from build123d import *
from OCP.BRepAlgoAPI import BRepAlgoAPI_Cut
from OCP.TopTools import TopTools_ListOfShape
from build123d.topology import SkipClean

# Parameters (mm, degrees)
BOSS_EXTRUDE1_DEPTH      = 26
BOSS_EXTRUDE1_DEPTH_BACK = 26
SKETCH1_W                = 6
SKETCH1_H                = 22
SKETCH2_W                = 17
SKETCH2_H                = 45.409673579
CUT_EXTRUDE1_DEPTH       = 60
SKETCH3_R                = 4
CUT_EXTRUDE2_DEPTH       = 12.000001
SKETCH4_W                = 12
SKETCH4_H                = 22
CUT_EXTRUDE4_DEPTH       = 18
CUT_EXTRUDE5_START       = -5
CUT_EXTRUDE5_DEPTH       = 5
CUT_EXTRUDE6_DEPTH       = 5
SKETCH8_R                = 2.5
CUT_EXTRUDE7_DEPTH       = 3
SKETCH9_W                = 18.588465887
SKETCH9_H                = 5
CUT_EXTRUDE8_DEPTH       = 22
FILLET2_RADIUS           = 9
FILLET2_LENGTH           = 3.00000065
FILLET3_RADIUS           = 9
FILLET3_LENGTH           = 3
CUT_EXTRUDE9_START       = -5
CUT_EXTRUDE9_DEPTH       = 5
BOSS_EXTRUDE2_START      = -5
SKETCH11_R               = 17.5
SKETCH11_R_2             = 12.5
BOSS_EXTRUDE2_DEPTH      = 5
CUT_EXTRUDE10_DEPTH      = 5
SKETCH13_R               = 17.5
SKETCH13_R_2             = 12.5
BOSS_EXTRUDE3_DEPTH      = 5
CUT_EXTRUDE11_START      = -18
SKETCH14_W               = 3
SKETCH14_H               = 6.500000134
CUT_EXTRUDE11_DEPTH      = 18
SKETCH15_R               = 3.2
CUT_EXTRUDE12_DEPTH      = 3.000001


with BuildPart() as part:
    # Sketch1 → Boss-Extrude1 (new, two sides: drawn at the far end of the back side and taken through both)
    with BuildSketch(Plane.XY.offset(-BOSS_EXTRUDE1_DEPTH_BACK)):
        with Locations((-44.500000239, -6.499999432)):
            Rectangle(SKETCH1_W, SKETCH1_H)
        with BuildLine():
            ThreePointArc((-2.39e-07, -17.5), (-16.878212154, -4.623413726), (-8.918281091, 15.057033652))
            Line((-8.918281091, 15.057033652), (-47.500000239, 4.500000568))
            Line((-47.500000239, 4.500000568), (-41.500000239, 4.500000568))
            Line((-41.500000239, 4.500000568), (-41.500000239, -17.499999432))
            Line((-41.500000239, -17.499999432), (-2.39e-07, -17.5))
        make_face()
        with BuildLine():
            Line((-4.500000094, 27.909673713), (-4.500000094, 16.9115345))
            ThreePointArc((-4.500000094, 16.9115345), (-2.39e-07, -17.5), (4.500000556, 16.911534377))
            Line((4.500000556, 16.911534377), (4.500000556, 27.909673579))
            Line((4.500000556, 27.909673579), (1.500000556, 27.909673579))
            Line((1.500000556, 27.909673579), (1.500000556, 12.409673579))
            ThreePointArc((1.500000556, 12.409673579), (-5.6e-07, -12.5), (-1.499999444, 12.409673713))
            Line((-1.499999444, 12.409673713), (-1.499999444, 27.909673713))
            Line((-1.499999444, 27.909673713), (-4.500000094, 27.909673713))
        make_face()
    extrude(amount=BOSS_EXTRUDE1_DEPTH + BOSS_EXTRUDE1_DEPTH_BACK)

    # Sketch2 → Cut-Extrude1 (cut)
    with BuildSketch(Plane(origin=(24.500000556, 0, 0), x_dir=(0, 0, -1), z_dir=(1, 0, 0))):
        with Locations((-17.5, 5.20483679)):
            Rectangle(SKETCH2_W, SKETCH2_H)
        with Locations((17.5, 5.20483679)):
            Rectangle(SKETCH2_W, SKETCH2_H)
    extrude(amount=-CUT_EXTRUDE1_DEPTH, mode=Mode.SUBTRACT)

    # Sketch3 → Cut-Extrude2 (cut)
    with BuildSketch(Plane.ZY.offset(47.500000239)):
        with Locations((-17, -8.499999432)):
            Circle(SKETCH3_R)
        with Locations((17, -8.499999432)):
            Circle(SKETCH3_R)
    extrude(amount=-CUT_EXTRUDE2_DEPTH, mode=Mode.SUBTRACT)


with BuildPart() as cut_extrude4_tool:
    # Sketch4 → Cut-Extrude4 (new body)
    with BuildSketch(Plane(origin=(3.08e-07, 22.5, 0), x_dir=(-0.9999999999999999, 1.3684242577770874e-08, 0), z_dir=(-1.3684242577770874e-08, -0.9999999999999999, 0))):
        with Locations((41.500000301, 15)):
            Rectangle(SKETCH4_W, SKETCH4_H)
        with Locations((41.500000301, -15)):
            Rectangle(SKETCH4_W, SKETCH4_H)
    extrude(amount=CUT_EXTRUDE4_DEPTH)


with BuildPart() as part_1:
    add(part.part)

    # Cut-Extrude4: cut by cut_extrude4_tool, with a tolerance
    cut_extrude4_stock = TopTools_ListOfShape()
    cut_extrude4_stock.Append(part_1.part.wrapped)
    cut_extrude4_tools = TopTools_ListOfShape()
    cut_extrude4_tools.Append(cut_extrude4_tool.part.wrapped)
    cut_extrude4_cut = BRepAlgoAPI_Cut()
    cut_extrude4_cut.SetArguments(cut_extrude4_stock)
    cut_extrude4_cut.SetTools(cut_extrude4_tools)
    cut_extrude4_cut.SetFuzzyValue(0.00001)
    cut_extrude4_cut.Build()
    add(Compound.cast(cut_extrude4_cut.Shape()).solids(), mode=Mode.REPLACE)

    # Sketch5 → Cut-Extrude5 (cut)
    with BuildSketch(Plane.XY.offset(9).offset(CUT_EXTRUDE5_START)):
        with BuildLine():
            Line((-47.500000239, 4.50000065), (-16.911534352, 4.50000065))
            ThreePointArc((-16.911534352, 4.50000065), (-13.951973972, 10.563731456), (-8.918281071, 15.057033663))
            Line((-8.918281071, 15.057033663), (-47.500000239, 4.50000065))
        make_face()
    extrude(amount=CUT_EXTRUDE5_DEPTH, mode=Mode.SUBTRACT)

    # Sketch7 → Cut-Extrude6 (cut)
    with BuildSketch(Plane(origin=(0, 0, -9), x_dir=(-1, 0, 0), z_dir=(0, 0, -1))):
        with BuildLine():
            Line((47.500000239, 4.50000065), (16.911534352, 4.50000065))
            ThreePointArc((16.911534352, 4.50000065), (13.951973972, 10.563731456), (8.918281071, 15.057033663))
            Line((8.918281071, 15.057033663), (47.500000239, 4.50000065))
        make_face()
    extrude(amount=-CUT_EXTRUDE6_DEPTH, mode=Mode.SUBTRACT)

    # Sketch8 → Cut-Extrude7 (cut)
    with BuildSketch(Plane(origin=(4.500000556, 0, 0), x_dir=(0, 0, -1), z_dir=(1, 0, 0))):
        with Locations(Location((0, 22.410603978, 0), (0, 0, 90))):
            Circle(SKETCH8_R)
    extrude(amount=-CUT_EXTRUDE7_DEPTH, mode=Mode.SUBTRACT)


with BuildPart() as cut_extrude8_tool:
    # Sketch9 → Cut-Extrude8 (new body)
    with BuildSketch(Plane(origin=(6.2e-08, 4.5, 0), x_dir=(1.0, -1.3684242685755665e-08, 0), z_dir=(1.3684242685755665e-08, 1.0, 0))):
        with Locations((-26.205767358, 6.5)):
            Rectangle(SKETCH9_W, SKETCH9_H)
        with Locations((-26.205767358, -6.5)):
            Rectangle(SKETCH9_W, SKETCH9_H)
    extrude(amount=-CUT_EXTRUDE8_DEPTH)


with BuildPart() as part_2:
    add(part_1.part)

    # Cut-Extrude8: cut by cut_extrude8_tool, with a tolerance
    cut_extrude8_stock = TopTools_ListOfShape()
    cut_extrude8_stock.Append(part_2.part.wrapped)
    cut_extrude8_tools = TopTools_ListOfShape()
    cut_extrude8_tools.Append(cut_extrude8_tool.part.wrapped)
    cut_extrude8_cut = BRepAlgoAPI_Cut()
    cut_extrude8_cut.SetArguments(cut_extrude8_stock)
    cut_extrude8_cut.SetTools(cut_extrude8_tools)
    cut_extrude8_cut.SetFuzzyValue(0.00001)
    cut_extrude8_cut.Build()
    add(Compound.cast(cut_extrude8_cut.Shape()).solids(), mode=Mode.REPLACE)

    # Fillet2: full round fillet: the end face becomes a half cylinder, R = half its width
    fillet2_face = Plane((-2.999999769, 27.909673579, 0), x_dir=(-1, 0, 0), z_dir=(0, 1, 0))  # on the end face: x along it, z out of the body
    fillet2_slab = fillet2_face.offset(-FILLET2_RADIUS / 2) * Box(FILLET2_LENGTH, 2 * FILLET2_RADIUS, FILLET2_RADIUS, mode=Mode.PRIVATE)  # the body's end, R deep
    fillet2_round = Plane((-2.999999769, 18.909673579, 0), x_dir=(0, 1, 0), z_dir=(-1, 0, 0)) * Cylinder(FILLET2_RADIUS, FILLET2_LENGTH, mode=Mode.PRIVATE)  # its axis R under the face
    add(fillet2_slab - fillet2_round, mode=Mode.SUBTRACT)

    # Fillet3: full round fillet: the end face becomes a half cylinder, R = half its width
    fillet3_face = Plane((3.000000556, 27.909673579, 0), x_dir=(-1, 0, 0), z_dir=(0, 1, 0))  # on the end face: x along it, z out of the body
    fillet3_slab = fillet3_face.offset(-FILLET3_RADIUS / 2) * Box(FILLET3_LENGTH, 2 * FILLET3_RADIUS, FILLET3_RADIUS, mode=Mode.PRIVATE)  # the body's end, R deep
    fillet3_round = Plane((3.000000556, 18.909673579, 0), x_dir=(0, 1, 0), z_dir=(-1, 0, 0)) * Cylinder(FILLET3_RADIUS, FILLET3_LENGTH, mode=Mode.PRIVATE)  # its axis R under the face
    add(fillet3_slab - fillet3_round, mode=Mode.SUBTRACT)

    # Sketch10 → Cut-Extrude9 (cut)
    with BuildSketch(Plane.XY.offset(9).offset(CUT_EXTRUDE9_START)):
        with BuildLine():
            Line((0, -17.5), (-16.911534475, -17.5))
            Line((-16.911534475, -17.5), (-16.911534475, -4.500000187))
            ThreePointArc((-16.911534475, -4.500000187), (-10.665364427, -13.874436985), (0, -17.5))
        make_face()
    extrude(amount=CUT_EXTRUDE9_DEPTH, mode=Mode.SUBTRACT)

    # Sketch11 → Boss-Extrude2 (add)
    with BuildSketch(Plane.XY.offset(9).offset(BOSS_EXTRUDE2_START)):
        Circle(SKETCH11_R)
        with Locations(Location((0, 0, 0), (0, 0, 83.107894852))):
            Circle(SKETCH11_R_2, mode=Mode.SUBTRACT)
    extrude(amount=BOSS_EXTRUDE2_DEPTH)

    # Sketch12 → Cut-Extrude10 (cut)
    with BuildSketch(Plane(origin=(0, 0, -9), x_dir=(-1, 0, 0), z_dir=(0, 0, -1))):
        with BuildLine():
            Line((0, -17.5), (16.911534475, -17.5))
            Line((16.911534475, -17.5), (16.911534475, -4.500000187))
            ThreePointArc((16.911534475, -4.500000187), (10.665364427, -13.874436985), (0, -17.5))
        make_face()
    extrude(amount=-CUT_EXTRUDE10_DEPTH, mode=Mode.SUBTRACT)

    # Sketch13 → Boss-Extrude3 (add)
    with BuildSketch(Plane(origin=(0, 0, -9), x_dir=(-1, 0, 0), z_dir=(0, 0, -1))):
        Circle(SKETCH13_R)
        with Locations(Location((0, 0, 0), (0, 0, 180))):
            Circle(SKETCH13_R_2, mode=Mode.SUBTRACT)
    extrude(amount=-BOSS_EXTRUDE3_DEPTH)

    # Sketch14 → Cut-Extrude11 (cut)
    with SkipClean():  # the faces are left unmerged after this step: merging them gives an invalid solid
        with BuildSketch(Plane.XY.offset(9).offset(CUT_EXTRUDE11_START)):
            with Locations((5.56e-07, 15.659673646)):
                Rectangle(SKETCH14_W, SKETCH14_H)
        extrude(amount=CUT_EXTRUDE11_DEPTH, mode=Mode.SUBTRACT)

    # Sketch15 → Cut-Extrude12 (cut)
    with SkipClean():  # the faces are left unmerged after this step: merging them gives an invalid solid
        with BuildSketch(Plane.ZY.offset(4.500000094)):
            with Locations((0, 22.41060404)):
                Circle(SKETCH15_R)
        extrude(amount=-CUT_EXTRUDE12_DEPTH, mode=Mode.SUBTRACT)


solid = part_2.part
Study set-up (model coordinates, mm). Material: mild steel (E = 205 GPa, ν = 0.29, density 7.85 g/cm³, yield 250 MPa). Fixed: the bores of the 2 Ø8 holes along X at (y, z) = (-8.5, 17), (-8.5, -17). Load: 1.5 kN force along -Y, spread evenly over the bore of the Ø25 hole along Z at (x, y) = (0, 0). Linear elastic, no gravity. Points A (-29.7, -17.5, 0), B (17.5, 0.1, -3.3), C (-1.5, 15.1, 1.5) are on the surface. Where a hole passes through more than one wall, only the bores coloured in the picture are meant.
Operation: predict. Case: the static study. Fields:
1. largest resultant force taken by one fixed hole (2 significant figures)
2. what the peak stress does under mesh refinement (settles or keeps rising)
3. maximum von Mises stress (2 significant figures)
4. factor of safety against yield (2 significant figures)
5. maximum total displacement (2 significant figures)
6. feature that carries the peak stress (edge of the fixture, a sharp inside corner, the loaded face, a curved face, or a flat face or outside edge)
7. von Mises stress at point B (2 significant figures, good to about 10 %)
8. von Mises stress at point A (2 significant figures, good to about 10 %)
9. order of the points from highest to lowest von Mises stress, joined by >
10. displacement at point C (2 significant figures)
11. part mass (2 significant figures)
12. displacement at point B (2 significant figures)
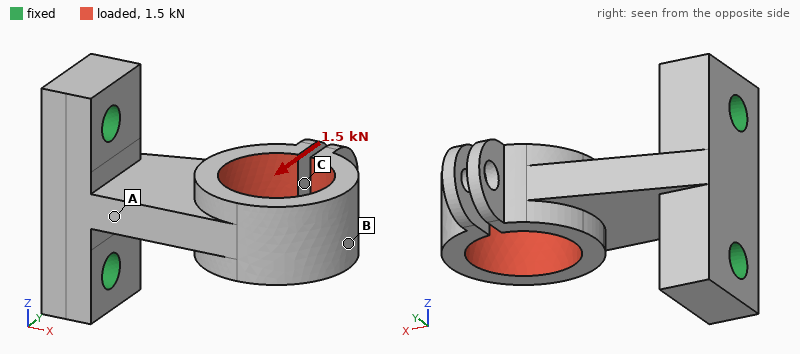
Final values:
780 N
settles
140 MPa
1.8
0.16 mm
a flat face or outside edge
22 MPa
55 MPa
A > B > C
0.042 mm
210 g
0.13 mm
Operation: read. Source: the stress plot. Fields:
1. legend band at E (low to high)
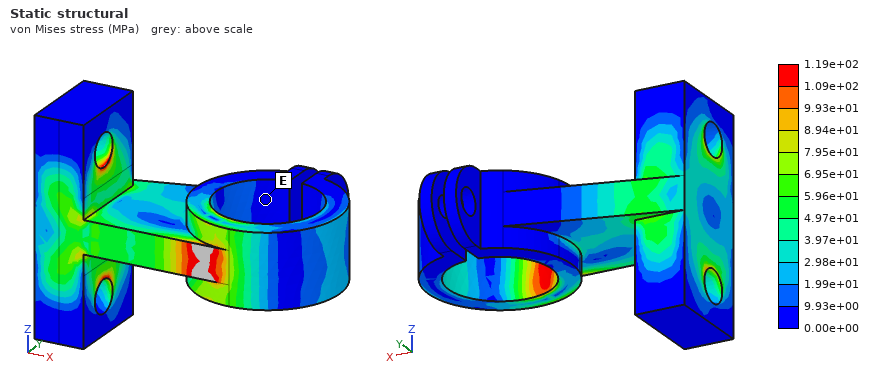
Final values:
0.00e+00 to 9.93e+00 MPa
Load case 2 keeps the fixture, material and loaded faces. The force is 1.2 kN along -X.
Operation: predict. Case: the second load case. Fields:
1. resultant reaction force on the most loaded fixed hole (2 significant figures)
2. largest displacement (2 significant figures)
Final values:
610 N
0.23 mm
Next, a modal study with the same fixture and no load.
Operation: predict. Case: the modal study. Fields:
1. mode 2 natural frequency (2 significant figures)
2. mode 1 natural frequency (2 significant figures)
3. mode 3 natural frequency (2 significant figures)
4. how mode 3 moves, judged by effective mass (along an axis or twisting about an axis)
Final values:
1500 Hz
1400 Hz
2900 Hz
along Y
